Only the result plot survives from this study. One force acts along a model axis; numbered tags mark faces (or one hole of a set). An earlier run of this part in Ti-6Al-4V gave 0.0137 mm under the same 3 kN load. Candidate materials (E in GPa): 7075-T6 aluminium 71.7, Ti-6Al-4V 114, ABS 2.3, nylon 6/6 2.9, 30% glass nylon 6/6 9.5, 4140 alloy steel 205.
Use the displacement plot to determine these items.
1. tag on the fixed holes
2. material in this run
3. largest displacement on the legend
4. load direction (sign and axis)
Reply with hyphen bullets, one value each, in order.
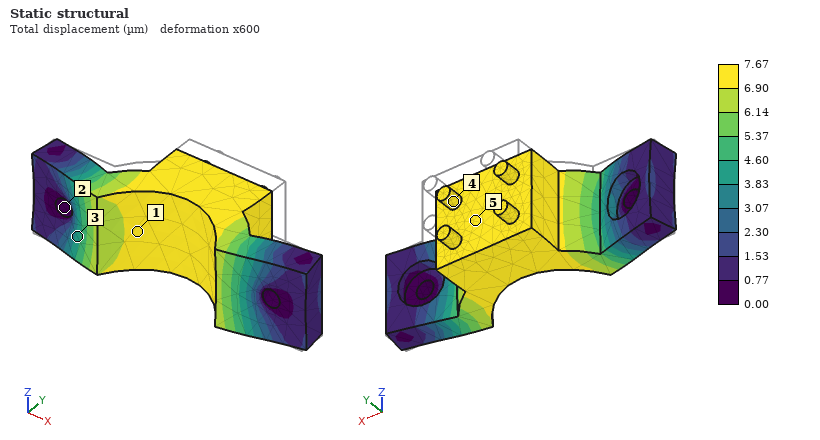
- 2
- 4140 alloy steel
- 7.67 µm
- -Y
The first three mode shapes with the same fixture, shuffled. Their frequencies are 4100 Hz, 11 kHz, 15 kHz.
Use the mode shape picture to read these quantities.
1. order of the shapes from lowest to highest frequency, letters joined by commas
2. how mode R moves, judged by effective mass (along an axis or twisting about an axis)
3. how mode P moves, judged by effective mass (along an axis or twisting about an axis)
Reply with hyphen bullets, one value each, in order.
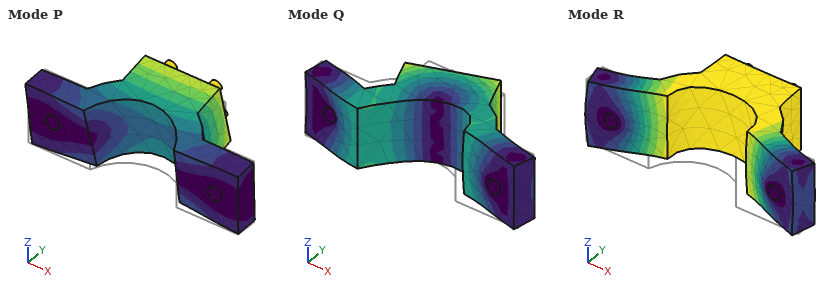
- P, R, Q
- along Y
- along Z
